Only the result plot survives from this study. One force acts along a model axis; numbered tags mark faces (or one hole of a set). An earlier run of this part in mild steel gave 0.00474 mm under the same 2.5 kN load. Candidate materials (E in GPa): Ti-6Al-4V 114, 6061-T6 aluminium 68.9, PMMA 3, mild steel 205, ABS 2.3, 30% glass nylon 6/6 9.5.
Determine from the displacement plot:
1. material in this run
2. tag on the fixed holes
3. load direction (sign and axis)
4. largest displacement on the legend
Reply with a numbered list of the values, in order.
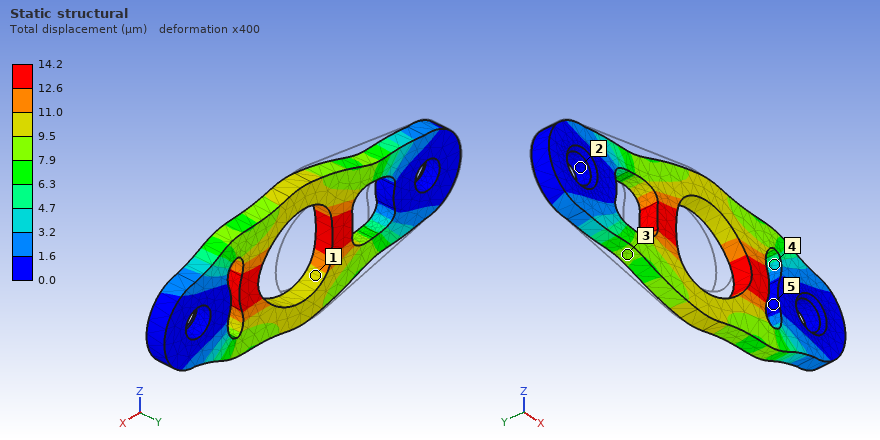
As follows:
1. 6061-T6 aluminium
2. 2
3. +X
4. 14.2 µm
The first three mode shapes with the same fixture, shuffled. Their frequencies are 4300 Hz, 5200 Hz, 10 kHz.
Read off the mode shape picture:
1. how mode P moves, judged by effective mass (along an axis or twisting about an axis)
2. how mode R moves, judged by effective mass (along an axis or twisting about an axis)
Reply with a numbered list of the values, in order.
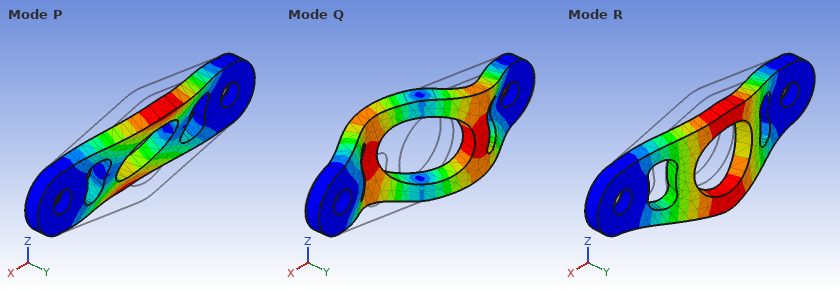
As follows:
1. twisting about X
2. along Y
